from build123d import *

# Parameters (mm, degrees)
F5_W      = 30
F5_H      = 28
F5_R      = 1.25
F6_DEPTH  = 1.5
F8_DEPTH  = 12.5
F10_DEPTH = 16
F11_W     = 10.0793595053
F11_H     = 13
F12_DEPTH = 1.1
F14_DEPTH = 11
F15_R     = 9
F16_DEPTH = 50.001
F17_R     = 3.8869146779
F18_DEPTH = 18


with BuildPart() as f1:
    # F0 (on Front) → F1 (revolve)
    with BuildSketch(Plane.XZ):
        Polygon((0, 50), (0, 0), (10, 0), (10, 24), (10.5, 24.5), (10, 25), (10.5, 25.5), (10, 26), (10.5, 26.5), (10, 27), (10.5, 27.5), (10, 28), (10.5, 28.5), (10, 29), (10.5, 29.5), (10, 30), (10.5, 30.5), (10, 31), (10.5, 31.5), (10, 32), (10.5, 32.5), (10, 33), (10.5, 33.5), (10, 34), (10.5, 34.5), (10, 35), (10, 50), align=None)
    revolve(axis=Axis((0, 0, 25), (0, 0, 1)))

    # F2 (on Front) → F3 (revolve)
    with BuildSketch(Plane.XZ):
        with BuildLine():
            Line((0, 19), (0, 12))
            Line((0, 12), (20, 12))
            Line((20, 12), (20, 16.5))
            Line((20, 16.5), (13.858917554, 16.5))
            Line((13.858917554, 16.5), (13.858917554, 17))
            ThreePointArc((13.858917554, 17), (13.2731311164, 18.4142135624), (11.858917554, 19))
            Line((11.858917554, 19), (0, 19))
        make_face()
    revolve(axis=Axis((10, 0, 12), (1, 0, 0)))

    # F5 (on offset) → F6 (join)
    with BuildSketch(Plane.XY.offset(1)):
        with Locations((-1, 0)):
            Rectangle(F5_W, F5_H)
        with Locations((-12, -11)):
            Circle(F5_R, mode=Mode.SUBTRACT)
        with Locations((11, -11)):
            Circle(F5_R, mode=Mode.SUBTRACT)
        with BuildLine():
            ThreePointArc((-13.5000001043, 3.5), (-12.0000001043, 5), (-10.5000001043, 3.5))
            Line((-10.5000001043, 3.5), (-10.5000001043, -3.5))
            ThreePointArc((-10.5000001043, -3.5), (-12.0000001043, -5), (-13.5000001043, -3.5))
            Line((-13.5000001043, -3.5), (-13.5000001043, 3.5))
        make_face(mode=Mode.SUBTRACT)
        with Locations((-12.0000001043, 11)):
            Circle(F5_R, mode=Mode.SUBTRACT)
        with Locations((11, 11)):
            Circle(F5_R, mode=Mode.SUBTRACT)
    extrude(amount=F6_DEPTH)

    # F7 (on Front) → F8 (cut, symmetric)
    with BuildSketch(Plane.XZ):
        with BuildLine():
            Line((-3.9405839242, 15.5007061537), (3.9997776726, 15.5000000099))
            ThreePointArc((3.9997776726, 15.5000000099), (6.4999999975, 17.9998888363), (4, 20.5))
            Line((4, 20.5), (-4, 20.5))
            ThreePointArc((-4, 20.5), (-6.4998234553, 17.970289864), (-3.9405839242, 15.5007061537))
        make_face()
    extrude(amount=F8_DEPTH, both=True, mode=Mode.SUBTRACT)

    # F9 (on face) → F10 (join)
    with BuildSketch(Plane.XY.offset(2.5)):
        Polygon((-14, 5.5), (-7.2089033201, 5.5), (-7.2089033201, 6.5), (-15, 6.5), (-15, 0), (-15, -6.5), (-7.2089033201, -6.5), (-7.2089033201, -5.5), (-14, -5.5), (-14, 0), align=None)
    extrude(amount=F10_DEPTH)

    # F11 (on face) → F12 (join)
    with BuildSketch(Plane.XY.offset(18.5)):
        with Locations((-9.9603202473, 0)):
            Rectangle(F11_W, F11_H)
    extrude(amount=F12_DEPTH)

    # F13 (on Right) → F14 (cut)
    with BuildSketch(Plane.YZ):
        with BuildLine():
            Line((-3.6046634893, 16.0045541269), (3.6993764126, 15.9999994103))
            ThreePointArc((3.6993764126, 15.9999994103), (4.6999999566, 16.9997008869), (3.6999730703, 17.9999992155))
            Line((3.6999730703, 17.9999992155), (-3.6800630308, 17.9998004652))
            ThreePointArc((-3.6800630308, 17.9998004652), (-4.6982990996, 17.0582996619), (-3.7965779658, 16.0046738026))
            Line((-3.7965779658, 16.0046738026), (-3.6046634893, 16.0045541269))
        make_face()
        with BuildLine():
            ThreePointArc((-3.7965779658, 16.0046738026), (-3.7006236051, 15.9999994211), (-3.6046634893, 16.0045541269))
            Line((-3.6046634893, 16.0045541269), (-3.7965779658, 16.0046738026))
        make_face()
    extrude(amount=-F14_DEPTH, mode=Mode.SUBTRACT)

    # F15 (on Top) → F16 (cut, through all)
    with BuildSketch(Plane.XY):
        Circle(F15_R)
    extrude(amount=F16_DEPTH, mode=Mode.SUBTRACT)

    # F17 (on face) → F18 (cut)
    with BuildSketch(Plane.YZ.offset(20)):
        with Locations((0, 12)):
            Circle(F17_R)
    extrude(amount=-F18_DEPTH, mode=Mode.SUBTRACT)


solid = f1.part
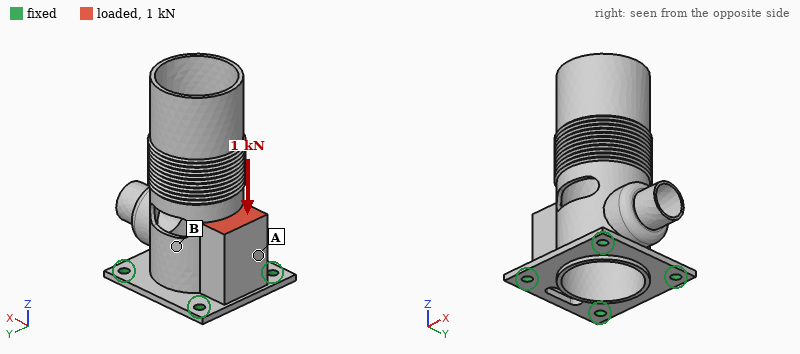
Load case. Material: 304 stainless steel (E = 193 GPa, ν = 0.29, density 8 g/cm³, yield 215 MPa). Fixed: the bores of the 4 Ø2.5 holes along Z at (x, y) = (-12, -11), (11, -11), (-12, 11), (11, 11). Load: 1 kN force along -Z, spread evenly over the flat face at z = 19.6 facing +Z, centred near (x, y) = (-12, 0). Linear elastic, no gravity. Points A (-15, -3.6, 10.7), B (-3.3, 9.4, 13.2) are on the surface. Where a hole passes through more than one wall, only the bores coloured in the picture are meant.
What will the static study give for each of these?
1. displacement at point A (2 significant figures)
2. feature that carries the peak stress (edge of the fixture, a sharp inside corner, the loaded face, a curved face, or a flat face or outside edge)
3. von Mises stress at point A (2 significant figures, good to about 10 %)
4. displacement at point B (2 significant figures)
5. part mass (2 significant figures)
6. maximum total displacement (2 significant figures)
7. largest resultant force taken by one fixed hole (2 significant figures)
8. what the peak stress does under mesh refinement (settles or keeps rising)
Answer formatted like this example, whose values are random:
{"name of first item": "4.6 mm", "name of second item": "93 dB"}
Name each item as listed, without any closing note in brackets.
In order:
{"displacement at point A": "20 µm", "feature that carries the peak stress": "edge of the fixture", "von Mises stress at point A": "38 MPa", "displacement at point B": "12 µm", "part mass": "38 g", "maximum total displacement": "45 µm", "largest resultant force taken by one fixed hole": "530 N", "what the peak stress does under mesh refinement": "keeps rising"}
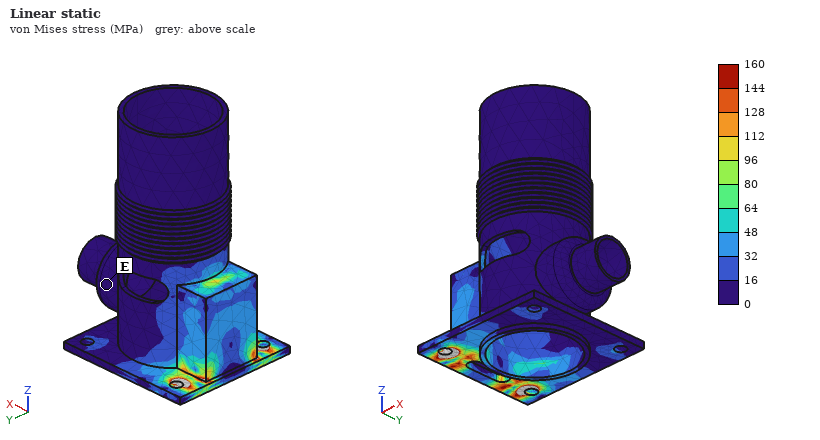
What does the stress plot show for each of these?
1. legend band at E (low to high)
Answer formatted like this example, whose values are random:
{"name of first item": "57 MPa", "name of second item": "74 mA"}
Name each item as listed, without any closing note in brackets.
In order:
{"legend band at E": "0 to 16 MPa"}
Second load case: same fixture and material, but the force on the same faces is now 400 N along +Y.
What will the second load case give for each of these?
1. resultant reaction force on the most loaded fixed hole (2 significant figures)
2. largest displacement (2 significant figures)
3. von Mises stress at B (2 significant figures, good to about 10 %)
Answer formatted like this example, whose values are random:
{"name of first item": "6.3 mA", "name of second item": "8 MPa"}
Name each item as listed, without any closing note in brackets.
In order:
{"resultant reaction force on the most loaded fixed hole": "340 N", "largest displacement": "48 µm", "von Mises stress at B": "26 MPa"}
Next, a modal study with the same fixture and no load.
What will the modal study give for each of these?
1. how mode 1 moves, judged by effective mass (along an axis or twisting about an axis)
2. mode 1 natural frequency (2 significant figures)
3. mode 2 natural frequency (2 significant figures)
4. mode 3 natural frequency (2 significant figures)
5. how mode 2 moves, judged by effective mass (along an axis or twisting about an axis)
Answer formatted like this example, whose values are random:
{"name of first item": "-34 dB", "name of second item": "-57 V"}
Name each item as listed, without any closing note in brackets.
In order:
{"how mode 1 moves, judged by effective mass": "along Y", "mode 1 natural frequency": "2700 Hz", "mode 2 natural frequency": "2900 Hz", "mode 3 natural frequency": "7700 Hz", "how mode 2 moves, judged by effective mass": "along X"}
